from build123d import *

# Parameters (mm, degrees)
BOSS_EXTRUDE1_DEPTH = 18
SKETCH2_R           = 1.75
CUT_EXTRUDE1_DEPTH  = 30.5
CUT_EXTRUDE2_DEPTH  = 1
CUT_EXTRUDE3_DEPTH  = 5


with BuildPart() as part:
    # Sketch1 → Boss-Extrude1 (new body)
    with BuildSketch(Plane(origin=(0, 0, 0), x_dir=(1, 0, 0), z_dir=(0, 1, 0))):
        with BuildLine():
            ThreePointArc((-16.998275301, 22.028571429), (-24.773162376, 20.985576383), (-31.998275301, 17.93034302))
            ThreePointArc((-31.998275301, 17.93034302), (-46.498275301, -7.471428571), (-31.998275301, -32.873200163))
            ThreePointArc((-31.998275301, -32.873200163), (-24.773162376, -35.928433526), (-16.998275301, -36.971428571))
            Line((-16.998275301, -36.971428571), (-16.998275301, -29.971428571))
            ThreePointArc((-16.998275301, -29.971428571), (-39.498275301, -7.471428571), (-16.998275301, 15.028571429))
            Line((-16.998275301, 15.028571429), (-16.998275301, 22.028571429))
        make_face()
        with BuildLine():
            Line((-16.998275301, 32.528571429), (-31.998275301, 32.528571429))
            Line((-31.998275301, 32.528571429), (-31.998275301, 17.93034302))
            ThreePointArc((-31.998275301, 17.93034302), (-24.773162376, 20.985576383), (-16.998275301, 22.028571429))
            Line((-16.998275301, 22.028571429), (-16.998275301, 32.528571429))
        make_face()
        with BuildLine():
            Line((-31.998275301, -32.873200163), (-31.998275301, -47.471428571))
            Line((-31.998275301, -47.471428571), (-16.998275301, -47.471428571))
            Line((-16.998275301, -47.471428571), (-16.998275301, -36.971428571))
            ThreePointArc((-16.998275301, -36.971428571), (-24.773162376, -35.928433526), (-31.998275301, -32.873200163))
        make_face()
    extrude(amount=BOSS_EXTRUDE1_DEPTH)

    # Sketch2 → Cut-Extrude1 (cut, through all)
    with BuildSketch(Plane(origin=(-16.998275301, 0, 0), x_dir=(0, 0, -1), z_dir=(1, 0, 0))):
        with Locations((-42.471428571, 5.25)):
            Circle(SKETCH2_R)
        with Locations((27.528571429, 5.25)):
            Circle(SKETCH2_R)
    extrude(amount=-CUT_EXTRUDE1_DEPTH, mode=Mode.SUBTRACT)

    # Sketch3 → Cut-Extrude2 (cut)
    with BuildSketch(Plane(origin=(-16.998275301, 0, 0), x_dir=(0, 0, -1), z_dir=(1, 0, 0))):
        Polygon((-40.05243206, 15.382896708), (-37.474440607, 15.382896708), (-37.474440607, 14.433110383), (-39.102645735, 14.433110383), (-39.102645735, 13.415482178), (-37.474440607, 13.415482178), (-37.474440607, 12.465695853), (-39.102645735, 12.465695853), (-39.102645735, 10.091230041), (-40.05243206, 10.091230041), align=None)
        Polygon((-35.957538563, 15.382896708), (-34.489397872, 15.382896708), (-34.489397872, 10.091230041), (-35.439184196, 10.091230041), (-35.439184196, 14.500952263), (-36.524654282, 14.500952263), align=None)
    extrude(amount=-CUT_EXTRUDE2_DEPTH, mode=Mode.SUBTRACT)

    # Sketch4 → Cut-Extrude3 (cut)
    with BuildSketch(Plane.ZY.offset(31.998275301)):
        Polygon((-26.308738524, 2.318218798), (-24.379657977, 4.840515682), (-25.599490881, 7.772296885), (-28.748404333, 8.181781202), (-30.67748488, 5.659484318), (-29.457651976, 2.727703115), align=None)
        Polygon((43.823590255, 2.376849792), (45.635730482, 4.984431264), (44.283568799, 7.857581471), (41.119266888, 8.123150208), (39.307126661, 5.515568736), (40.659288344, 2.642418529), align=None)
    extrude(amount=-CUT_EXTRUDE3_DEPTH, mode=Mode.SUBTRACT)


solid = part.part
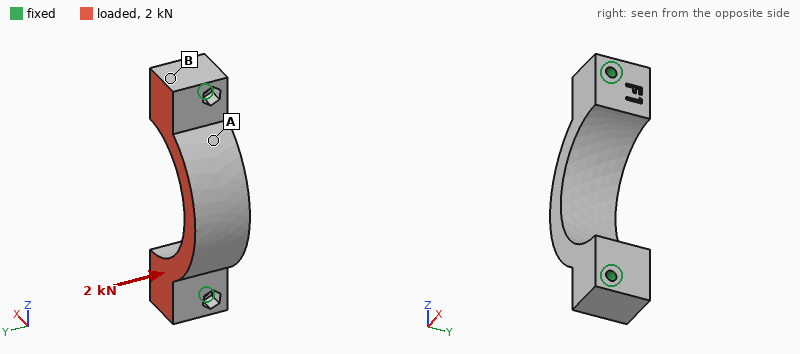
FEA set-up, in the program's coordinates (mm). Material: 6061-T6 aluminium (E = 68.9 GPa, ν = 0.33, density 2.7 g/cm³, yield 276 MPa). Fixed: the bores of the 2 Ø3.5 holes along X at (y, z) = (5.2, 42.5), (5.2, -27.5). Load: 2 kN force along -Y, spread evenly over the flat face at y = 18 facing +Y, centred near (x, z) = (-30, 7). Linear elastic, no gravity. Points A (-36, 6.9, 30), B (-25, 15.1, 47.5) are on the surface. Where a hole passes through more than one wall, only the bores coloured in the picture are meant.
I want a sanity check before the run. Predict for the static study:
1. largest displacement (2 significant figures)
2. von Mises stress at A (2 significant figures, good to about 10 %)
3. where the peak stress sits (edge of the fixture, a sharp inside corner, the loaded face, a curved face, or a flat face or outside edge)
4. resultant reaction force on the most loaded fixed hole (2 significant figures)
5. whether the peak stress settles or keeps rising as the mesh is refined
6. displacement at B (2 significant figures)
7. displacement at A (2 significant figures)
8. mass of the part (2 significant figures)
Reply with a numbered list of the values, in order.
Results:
1. 47 µm
2. 19 MPa
3. edge of the fixture
4. 1.0 kN
5. keeps rising
6. 8.2 µm
7. 21 µm
8. 44 g
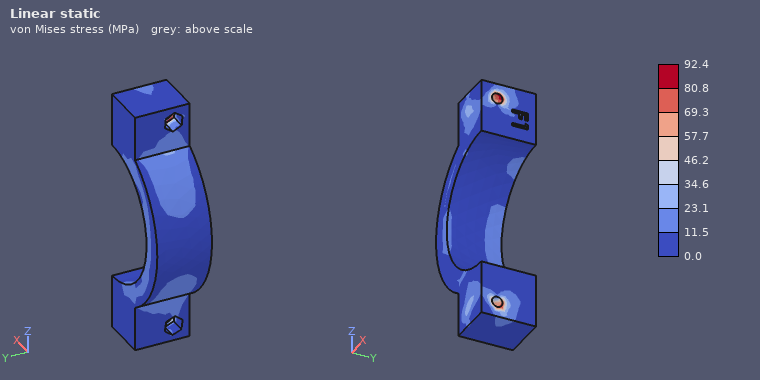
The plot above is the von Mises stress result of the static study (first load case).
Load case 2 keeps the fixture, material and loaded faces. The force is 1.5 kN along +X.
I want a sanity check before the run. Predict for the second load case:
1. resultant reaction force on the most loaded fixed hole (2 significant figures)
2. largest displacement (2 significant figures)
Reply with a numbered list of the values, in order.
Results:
1. 800 N
2. 30 µm
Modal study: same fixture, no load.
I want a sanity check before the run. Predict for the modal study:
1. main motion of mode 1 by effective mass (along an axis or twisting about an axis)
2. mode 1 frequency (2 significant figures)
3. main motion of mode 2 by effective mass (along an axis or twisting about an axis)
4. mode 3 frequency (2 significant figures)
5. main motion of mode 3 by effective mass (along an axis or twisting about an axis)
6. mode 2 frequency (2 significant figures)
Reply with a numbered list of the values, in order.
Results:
1. along Y
2. 6100 Hz
3. along Z
4. 16 kHz
5. along X
6. 13 kHz
